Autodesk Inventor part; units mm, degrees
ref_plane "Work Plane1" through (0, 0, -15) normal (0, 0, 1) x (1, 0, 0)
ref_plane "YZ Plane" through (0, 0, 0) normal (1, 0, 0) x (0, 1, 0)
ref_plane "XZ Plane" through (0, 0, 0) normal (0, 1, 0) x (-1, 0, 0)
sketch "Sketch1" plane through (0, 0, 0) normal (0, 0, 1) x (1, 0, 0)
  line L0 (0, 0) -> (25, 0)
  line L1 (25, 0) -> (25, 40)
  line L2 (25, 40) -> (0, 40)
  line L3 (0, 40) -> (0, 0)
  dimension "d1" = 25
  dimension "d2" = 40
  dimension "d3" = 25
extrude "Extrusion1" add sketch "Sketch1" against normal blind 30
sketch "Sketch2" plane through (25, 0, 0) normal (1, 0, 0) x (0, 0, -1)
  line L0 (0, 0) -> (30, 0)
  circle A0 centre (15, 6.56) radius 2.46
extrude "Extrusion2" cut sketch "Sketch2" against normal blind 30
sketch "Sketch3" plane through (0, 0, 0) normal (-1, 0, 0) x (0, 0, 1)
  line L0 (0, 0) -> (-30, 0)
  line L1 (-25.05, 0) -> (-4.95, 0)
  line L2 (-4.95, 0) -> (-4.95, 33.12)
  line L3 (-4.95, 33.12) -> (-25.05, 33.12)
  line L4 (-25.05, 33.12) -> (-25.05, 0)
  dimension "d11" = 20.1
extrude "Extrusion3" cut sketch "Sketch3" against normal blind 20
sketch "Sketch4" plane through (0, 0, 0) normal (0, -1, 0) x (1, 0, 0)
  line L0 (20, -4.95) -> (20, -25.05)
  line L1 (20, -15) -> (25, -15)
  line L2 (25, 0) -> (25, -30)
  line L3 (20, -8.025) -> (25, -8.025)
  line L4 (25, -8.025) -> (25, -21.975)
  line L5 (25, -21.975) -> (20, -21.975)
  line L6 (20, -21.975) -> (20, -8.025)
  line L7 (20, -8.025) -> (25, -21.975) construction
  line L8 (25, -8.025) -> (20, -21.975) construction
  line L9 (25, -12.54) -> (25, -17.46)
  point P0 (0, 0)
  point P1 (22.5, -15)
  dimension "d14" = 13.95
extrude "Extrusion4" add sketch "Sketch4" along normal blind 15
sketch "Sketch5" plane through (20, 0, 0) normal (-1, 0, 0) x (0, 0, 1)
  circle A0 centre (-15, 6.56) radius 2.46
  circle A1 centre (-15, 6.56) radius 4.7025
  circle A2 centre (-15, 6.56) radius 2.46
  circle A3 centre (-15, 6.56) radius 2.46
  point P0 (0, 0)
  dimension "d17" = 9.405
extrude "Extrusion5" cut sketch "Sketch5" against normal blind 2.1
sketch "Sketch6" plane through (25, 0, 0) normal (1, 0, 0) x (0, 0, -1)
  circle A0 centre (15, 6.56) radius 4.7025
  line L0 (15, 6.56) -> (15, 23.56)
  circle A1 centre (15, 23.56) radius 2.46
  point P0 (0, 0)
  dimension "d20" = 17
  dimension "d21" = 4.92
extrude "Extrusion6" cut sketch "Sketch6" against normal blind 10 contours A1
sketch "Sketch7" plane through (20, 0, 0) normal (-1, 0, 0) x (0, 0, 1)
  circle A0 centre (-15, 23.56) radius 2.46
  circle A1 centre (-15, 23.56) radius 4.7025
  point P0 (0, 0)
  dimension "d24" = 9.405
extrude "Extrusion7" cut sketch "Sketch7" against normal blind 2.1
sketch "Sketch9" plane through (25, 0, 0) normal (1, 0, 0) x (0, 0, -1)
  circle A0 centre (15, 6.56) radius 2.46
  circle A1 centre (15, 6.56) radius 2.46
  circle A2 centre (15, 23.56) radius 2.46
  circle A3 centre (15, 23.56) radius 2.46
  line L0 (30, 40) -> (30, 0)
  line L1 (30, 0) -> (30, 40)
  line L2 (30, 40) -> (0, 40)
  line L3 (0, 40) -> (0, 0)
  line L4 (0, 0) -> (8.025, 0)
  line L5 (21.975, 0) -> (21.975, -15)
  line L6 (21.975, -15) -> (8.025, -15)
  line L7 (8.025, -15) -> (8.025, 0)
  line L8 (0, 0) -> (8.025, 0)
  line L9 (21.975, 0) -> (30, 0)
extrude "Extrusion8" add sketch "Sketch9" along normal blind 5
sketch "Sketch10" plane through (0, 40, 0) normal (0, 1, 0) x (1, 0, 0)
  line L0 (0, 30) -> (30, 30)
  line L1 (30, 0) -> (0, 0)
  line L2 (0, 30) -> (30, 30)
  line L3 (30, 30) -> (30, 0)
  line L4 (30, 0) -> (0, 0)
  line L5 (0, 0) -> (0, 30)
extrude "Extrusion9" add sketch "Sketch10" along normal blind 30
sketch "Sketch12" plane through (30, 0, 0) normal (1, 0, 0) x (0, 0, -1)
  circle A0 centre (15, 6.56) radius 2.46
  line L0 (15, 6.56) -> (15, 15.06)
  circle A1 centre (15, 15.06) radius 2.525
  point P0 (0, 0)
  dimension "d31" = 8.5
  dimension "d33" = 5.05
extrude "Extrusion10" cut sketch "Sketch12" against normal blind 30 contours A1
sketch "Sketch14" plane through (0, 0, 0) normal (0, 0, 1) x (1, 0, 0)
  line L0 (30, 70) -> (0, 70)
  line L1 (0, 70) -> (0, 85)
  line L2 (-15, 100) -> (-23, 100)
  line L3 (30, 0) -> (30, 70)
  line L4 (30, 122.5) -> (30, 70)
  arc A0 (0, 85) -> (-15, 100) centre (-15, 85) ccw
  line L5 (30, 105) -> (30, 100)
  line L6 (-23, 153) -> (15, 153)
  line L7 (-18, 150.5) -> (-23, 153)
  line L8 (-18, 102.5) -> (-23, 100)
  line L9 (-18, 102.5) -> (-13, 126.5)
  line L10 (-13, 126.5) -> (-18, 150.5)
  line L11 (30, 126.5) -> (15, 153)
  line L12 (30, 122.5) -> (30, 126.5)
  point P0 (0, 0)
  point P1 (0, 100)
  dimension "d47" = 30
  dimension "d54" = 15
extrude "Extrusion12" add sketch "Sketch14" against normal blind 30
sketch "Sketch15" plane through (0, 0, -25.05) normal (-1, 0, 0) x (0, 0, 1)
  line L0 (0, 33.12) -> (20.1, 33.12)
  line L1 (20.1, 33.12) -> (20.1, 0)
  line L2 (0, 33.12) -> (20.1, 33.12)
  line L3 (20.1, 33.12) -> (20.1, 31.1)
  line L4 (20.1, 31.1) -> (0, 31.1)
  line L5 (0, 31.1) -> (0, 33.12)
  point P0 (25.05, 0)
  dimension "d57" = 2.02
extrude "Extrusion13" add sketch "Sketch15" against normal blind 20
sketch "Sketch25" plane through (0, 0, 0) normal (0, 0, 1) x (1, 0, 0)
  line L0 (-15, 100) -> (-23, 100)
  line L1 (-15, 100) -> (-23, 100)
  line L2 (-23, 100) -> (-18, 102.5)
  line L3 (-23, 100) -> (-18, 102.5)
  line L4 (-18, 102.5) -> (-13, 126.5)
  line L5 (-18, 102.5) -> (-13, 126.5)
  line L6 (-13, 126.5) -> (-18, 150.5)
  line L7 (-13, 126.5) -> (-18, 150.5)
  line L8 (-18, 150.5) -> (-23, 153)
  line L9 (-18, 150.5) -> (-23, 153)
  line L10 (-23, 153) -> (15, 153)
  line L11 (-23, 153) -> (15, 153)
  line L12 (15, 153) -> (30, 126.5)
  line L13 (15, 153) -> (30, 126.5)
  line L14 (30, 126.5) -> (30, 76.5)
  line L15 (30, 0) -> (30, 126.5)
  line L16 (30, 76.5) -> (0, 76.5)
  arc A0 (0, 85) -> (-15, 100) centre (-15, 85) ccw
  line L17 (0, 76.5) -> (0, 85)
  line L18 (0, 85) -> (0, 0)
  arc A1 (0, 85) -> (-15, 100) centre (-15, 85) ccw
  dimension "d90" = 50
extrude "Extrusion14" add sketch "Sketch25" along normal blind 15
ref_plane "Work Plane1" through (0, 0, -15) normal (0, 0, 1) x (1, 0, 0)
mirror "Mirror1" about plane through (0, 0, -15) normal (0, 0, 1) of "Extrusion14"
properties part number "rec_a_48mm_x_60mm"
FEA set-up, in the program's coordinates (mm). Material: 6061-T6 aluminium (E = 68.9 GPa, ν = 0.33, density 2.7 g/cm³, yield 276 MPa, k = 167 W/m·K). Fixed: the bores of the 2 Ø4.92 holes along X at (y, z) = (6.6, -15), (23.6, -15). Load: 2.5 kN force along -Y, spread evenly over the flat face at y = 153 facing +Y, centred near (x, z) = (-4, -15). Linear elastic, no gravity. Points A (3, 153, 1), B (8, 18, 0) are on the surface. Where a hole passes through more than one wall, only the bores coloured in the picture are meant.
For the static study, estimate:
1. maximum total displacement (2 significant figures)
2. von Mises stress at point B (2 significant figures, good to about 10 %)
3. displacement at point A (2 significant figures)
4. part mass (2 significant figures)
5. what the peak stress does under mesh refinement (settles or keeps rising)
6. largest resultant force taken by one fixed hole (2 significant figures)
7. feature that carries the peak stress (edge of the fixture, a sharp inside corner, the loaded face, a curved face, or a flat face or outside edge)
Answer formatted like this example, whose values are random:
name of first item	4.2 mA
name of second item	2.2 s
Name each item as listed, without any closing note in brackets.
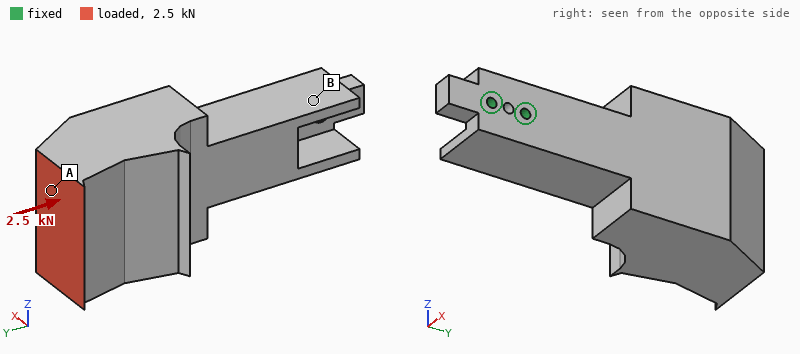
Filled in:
maximum total displacement	0.29 mm
von Mises stress at point B	19 MPa
displacement at point A	0.27 mm
part mass	640 g
what the peak stress does under mesh refinement	keeps rising
largest resultant force taken by one fixed hole	3.4 kN
feature that carries the peak stress	edge of the fixture
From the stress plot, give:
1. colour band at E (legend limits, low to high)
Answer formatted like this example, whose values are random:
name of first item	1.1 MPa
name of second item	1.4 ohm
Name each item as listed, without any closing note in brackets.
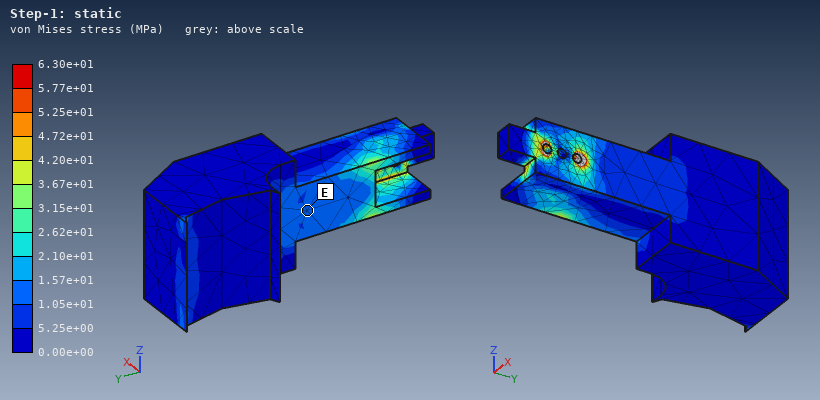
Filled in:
colour band at E	1.05e+01 to 1.57e+01 MPa
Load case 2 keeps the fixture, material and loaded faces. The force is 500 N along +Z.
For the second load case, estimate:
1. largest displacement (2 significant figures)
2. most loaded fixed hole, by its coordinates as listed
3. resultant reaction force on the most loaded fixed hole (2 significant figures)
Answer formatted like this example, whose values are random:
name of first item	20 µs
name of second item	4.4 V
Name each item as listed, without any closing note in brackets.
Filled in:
largest displacement	0.21 mm
most loaded fixed hole, by its coordinates as listed	(23.6, -15)
resultant reaction force on the most loaded fixed hole	3.3 kN
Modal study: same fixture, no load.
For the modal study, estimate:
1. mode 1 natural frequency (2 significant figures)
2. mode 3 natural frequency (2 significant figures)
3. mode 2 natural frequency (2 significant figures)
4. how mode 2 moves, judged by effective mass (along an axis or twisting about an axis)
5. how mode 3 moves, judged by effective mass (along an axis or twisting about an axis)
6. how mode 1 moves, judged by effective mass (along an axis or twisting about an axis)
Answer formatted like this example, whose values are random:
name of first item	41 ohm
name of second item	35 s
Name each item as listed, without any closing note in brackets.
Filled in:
mode 1 natural frequency	440 Hz
mode 3 natural frequency	1300 Hz
mode 2 natural frequency	510 Hz
how mode 2 moves, judged by effective mass	along Z
how mode 3 moves, judged by effective mass	twisting about Y
how mode 1 moves, judged by effective mass	along X
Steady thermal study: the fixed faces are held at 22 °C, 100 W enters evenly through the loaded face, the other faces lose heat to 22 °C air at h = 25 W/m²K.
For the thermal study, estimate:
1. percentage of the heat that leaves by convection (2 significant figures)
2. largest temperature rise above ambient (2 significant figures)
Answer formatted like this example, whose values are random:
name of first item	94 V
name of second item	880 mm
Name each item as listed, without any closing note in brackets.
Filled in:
percentage of the heat that leaves by convection	28 %
largest temperature rise above ambient	66 K
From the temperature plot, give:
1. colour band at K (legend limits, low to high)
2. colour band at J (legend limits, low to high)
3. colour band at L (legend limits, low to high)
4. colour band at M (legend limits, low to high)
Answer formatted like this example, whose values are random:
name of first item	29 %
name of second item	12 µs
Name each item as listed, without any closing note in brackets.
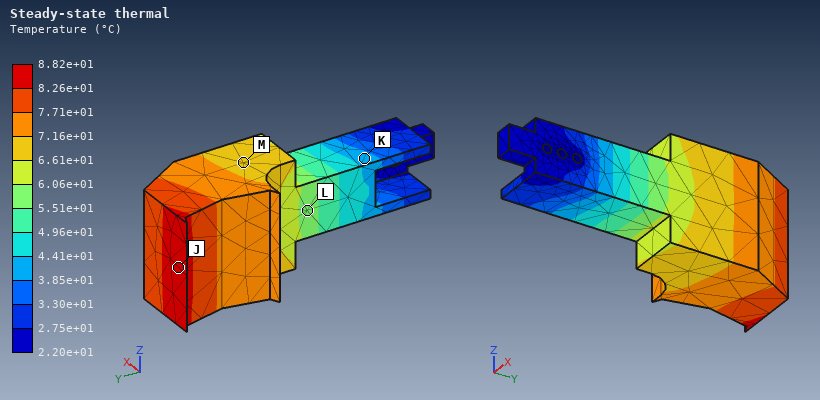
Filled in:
colour band at K	3.85e+01 to 4.41e+01 °C
colour band at J	8.26e+01 to 8.82e+01 °C
colour band at L	5.51e+01 to 6.06e+01 °C
colour band at M	6.61e+01 to 7.16e+01 °C
